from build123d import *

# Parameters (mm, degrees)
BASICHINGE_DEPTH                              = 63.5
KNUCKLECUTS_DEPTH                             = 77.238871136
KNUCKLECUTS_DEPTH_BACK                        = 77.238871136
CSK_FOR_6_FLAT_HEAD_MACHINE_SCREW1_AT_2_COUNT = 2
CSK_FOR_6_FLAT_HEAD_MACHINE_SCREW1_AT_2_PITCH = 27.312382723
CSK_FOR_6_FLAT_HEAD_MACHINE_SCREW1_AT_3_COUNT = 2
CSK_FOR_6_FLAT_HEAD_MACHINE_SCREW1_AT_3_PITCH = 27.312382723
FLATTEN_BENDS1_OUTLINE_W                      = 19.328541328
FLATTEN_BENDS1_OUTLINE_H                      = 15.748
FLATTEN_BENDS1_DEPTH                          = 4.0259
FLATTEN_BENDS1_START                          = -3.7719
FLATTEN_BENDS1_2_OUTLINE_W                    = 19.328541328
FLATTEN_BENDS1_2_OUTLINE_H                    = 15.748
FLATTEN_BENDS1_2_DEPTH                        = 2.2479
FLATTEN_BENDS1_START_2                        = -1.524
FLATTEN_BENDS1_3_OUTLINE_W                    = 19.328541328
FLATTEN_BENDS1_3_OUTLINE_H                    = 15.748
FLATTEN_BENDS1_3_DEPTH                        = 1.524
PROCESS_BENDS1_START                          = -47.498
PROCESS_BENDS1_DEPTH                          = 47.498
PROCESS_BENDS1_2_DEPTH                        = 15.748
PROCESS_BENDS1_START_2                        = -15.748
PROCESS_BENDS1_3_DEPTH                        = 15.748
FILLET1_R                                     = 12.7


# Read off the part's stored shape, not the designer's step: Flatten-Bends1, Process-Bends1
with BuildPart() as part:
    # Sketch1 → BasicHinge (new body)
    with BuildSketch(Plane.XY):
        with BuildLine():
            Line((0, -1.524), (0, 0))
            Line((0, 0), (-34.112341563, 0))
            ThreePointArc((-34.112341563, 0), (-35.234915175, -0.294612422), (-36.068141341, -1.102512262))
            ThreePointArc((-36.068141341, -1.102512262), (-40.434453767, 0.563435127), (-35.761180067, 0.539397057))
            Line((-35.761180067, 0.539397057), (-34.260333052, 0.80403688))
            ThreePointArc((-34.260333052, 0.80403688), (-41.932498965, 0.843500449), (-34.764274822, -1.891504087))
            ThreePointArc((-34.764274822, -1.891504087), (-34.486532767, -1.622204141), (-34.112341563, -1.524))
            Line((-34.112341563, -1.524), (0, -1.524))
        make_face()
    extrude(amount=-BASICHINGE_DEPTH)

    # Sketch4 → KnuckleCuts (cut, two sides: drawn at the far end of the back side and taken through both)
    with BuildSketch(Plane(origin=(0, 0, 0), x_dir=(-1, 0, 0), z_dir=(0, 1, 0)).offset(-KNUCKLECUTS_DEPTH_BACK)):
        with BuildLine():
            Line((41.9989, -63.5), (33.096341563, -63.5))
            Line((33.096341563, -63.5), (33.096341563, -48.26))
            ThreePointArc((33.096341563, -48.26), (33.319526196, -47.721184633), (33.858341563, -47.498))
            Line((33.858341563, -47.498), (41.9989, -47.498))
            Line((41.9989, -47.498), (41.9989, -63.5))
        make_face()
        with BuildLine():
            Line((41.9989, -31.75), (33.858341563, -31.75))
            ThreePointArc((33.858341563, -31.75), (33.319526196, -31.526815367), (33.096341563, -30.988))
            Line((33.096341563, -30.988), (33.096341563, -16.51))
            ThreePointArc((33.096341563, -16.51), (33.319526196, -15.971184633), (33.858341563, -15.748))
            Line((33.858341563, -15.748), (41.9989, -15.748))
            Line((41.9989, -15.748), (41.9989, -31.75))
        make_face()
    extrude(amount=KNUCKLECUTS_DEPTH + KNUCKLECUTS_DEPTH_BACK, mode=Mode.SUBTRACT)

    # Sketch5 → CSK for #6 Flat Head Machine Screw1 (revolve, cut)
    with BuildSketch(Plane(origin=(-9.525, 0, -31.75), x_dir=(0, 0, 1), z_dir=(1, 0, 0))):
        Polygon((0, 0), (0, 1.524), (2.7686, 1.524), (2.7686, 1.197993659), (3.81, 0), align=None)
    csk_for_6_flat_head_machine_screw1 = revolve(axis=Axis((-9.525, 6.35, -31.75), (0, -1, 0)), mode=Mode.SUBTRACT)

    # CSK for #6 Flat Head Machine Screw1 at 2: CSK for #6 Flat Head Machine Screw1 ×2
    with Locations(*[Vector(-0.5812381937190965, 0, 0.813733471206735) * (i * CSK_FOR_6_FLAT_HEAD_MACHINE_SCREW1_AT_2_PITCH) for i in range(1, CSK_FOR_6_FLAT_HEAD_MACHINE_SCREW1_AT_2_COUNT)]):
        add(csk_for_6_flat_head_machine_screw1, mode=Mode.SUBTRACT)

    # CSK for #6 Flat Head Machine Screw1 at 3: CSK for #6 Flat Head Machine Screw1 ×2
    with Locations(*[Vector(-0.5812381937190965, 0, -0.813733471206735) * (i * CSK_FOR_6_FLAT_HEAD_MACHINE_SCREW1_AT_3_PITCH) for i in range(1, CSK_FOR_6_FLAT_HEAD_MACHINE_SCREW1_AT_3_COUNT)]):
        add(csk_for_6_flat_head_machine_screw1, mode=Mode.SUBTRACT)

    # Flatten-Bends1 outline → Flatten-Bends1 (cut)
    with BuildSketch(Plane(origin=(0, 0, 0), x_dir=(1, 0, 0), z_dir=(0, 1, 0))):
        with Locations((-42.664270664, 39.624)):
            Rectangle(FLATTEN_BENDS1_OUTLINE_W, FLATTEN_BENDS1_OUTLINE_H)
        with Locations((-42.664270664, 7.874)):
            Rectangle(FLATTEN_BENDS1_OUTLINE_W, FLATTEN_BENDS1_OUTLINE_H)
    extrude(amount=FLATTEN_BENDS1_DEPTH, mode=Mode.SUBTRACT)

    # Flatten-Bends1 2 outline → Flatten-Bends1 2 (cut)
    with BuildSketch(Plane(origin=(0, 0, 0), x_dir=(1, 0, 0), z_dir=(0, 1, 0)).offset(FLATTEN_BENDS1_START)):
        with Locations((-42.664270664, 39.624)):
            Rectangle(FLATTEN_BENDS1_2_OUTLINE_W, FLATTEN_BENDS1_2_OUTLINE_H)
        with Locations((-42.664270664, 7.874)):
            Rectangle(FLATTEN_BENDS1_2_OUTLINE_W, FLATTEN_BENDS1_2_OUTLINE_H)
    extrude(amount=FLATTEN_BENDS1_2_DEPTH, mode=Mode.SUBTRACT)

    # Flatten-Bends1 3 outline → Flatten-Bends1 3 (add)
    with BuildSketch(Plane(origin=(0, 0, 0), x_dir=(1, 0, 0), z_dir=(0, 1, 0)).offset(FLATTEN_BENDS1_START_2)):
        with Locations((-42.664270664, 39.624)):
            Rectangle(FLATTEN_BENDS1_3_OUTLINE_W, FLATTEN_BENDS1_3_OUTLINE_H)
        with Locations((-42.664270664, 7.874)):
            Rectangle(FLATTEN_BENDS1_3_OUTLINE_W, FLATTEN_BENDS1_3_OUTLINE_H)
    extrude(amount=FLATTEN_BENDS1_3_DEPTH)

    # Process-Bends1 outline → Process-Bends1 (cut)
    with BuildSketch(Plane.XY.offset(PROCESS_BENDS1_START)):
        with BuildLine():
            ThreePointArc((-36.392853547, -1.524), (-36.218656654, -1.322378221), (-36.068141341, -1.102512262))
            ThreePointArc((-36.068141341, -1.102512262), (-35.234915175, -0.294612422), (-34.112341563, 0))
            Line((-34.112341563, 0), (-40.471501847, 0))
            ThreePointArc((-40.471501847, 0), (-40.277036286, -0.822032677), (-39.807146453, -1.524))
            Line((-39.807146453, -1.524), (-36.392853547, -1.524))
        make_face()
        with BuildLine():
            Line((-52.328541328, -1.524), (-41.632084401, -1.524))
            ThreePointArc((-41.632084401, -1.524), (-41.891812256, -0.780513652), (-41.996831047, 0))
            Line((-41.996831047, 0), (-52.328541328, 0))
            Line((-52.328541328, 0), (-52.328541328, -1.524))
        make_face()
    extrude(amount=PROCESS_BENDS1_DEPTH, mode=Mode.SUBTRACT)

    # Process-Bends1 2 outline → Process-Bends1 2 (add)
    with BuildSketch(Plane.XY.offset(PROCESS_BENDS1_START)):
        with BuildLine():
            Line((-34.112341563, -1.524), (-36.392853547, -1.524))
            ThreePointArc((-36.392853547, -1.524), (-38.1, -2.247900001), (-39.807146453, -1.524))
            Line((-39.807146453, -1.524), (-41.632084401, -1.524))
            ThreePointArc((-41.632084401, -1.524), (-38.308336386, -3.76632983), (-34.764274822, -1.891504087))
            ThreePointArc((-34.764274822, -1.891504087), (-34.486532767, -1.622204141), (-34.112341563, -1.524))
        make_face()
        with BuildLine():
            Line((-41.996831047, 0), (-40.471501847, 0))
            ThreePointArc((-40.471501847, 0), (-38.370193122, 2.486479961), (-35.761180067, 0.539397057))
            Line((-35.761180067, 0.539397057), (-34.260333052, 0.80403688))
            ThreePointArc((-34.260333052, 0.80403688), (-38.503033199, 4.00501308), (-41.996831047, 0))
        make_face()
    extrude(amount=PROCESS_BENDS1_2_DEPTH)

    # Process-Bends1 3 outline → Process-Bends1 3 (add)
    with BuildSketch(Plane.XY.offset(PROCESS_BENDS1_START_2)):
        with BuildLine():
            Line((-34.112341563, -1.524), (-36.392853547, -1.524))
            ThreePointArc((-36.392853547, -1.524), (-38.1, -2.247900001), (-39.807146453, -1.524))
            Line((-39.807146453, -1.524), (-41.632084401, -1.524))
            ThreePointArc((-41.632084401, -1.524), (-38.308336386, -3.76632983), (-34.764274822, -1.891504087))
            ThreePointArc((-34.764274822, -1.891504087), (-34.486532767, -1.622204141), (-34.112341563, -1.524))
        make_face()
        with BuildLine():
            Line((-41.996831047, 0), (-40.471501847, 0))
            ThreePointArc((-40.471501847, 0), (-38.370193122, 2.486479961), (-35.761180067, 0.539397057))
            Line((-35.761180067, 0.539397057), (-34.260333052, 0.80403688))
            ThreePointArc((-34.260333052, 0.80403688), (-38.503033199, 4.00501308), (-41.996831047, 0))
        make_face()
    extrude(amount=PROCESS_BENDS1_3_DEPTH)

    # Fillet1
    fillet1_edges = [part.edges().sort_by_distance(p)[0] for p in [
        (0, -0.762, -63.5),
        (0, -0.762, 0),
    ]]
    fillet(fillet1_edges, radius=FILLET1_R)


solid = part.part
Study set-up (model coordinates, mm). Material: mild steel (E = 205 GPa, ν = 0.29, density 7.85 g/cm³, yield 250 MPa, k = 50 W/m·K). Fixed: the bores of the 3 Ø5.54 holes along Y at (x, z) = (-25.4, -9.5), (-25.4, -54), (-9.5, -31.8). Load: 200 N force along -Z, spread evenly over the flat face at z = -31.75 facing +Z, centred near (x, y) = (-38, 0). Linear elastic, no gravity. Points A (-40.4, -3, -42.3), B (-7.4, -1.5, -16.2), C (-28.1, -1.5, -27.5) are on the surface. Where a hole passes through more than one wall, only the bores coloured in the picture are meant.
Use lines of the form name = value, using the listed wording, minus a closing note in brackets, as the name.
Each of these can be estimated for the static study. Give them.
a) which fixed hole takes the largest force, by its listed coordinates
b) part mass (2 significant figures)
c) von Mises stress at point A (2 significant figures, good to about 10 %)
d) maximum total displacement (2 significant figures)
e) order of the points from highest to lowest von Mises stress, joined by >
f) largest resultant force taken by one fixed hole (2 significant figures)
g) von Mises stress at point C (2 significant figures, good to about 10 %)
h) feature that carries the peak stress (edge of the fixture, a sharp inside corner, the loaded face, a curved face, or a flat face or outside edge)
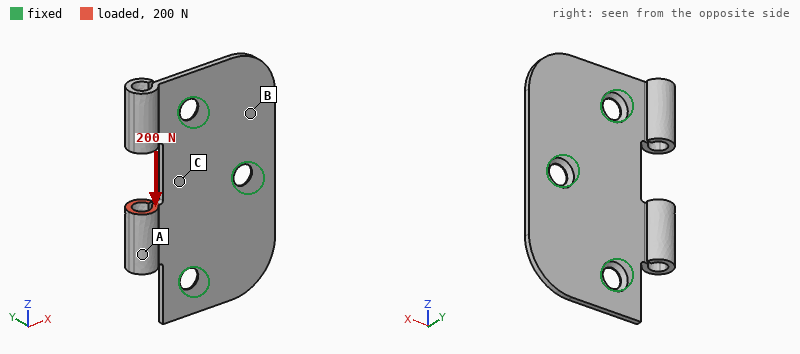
which fixed hole takes the largest force, by its listed coordinates = (-25.4, -54)
part mass = 31 g
von Mises stress at point A = 43 MPa
maximum total displacement = 33 µm
order of the points from highest to lowest von Mises stress, joined by > = A > C > B
largest resultant force taken by one fixed hole = 140 N
von Mises stress at point C = 15 MPa
feature that carries the peak stress = a curved face
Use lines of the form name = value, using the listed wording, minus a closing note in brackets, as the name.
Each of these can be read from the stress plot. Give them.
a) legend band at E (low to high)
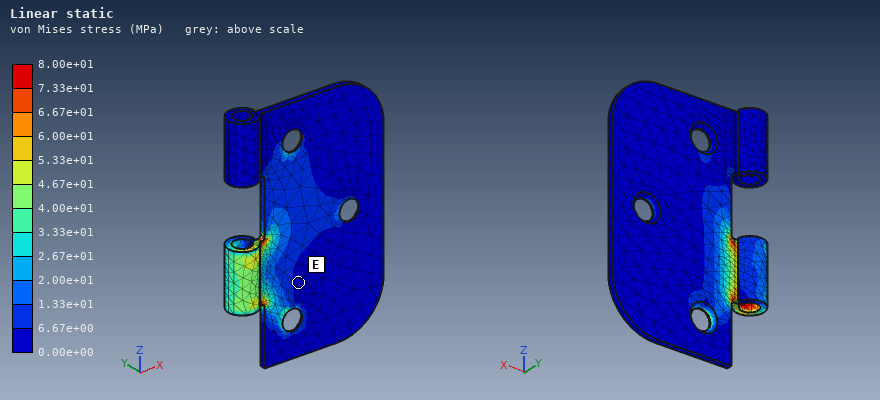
legend band at E = 0.00e+00 to 6.67e+00 MPa
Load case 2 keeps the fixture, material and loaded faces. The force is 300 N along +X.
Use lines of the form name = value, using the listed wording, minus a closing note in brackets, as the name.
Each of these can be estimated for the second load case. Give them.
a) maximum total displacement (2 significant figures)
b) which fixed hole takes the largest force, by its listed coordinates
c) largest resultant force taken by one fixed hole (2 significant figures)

maximum total displacement = 75 µm
which fixed hole takes the largest force, by its listed coordinates = (-9.5, -31.8)
largest resultant force taken by one fixed hole = 200 N
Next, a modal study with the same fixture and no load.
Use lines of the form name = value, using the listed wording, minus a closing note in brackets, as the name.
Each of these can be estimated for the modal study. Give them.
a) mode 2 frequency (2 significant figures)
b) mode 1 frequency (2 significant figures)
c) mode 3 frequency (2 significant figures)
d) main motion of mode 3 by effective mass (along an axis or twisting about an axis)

mode 2 frequency = 2800 Hz
mode 1 frequency = 2300 Hz
mode 3 frequency = 3400 Hz
main motion of mode 3 by effective mass = twisting about X
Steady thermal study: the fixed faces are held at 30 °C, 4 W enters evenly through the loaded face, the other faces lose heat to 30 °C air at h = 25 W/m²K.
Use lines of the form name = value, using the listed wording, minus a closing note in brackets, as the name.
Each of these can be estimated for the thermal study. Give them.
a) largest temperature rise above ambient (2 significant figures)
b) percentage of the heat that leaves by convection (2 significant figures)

largest temperature rise above ambient = 65 K
percentage of the heat that leaves by convection = 29 %
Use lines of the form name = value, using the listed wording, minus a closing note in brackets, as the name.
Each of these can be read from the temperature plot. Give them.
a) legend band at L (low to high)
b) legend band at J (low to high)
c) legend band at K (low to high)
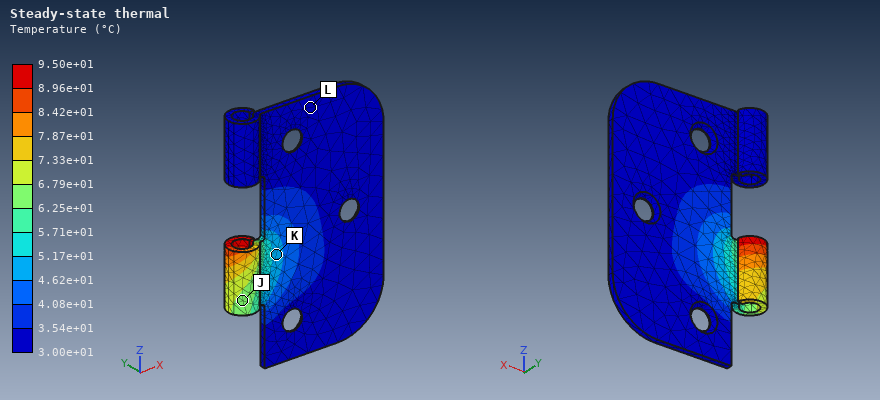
legend band at L = 3.00e+01 to 3.54e+01 °C
legend band at J = 6.25e+01 to 6.79e+01 °C
legend band at K = 4.62e+01 to 5.17e+01 °C
